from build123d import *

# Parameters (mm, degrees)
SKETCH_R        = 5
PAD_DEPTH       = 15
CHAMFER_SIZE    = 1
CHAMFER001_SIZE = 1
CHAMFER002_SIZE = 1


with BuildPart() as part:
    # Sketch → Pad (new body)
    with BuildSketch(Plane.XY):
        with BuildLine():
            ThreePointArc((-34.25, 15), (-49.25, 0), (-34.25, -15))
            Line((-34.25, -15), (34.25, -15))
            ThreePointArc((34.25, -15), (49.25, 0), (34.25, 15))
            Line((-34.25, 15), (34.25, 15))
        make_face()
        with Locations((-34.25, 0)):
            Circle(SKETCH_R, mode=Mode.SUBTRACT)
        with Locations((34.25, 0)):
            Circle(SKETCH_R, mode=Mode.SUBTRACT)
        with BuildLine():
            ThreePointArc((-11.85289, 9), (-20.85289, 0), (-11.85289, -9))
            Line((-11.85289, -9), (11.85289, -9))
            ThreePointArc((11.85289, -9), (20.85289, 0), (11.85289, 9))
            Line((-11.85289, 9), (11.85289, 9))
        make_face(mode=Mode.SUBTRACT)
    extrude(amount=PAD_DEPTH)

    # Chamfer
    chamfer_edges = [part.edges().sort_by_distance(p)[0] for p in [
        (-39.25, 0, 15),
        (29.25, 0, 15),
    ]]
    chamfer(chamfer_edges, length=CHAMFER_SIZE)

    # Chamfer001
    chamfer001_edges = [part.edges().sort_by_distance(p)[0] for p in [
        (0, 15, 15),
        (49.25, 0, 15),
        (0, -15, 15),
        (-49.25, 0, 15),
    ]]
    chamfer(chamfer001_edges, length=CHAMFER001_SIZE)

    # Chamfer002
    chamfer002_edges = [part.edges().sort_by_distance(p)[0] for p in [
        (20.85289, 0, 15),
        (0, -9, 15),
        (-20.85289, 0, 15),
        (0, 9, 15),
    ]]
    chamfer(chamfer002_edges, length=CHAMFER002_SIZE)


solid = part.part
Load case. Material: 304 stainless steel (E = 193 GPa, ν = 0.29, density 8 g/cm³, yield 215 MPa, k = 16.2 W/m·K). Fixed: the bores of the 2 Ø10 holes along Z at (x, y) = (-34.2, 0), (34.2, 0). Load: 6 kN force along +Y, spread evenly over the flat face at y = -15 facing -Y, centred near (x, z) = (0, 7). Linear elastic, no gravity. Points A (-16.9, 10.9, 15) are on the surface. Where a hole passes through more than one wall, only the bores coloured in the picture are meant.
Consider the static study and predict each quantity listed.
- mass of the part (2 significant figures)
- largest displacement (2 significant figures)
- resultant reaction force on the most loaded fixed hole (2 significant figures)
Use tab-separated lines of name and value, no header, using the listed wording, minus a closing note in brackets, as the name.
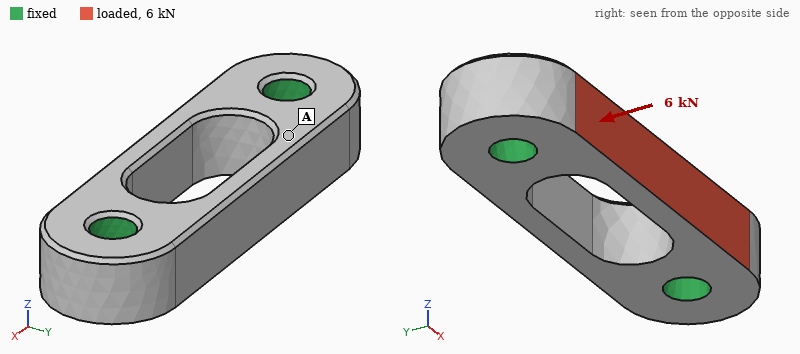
mass of the part	230 g
largest displacement	17 µm
resultant reaction force on the most loaded fixed hole	3.3 kN
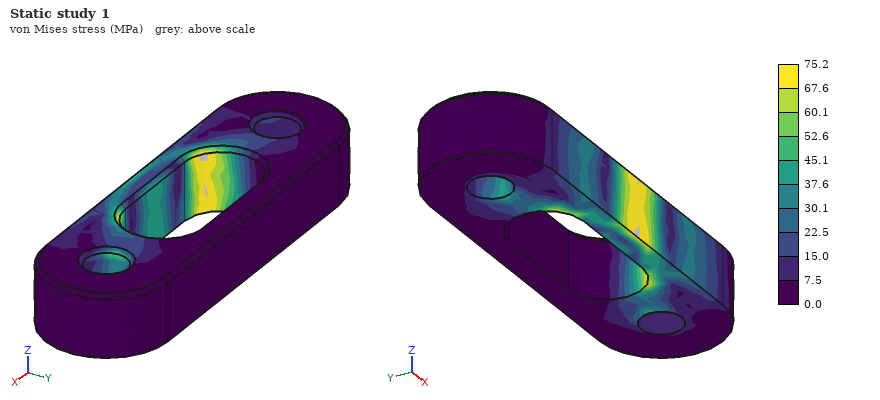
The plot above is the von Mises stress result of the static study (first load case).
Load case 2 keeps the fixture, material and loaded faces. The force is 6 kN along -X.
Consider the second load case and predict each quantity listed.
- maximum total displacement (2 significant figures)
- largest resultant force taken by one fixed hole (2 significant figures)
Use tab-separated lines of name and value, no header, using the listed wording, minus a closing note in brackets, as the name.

maximum total displacement	4.0 µm
largest resultant force taken by one fixed hole	3.0 kN
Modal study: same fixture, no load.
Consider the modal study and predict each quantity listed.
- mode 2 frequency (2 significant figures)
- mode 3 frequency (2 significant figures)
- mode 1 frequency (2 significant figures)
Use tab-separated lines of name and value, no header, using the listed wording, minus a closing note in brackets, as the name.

mode 2 frequency	16 kHz
mode 3 frequency	16 kHz
mode 1 frequency	15 kHz
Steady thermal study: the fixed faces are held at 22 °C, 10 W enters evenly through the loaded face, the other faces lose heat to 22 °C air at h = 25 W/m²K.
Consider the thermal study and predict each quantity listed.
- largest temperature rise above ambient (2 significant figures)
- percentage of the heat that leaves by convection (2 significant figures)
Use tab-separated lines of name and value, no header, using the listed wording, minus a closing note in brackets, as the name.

largest temperature rise above ambient	33 K
percentage of the heat that leaves by convection	10 %
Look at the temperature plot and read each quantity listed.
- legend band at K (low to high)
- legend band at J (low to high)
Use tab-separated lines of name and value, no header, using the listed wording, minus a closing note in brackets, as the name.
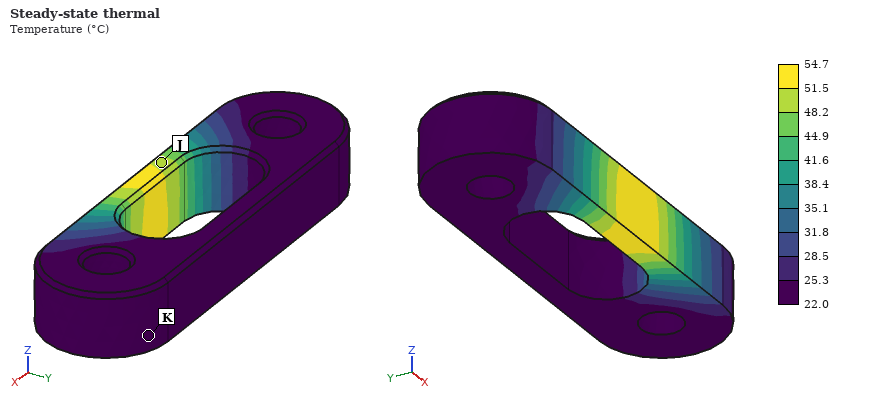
legend band at K	22.0 to 25.3 °C
legend band at J	48.2 to 51.5 °C
